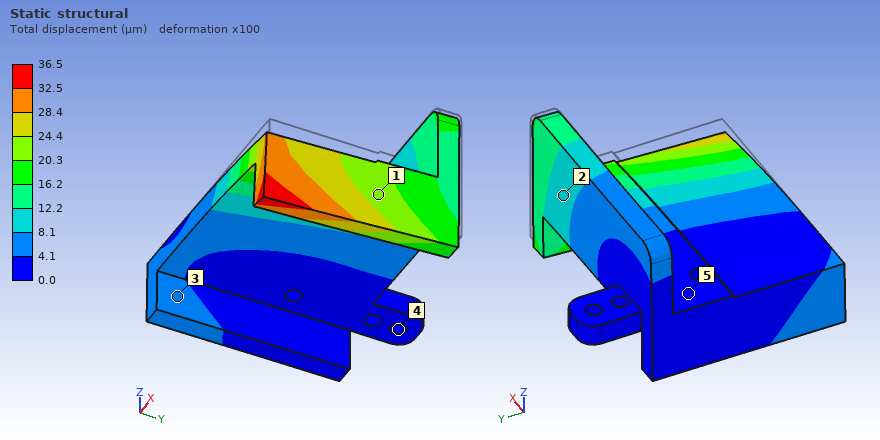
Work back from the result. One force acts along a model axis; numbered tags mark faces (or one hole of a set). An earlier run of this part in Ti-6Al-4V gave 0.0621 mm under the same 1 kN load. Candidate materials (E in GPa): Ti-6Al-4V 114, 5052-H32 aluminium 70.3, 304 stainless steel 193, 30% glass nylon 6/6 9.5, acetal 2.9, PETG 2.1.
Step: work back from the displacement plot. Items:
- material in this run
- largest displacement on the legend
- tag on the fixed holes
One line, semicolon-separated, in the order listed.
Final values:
304 stainless steel; 36.5 µm; 4
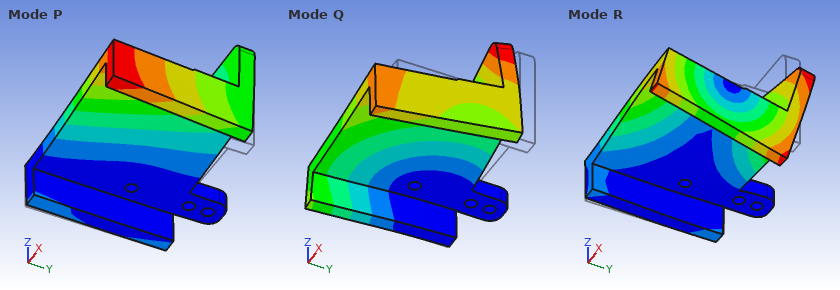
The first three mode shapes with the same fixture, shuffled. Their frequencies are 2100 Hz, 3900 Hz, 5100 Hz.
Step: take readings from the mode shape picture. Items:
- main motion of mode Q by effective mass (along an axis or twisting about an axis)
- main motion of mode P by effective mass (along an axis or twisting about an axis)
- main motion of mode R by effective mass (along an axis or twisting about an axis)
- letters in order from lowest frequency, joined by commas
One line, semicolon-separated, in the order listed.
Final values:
along Y; along Z; twisting about X; P, R, Q
